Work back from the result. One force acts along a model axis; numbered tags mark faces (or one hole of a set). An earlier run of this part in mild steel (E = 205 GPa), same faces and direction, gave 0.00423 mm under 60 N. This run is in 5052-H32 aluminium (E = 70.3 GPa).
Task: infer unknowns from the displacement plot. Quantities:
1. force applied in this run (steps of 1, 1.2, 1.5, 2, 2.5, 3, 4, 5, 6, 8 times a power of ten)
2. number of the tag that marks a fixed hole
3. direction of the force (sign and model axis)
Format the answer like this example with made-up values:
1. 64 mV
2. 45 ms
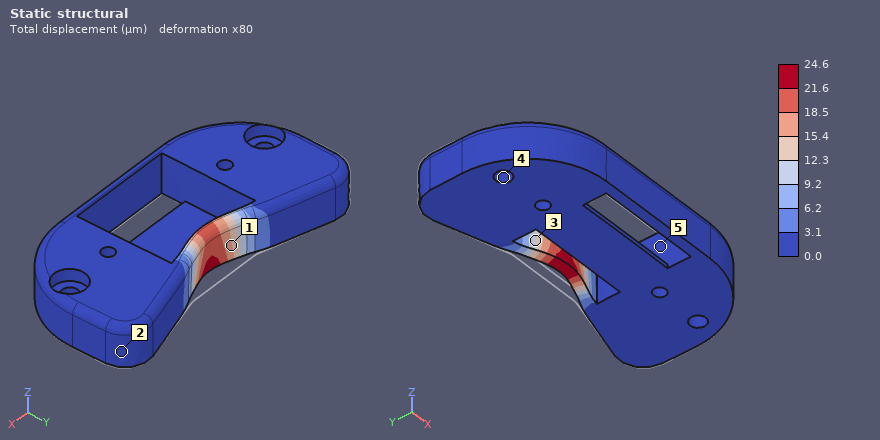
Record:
1. 120 N
2. 4
3. -Y
